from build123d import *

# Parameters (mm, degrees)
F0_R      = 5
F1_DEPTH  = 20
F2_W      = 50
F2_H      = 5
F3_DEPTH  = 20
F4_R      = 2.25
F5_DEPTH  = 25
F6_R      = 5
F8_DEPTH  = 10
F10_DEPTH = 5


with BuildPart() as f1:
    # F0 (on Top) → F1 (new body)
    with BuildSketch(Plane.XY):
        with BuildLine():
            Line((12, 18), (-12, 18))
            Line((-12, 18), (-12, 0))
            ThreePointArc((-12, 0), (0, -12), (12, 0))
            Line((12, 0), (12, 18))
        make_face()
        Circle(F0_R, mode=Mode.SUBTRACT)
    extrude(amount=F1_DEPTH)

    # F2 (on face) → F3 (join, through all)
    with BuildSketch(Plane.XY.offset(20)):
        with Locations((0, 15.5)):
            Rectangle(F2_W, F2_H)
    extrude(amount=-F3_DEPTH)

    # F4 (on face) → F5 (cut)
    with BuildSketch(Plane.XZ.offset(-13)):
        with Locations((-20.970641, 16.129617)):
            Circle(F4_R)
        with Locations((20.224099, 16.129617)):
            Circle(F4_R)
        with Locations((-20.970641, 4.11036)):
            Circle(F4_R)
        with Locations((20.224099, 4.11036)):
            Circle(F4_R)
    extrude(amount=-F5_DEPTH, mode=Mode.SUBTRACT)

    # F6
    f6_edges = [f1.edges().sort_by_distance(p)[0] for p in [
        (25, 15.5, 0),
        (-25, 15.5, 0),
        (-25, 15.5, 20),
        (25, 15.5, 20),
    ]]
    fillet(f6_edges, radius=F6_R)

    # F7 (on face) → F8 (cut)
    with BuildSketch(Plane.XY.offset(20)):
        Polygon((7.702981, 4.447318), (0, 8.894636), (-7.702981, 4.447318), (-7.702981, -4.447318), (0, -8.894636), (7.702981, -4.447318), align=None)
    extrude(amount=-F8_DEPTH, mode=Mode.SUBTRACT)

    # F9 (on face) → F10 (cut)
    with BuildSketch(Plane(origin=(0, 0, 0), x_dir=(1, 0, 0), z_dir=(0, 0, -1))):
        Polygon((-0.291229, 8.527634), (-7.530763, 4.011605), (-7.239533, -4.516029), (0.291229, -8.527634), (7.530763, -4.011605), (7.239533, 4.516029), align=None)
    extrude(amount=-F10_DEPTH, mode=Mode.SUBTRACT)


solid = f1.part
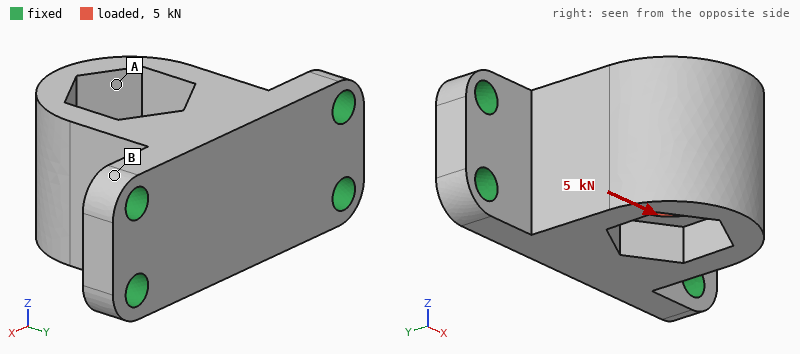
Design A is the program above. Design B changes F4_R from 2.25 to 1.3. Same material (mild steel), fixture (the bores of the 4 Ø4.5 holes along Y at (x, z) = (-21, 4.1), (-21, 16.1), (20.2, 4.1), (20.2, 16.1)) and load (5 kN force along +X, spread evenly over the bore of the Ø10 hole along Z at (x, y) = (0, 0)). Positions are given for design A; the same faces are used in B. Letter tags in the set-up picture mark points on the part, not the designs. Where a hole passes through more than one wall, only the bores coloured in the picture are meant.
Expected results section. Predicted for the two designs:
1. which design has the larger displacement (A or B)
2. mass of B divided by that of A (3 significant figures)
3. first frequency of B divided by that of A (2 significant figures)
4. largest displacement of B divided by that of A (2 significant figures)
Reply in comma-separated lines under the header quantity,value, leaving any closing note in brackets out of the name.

quantity,value
which design has the larger displacement,B
mass of B divided by that of A,1.02
first frequency of B divided by that of A,0.91
largest displacement of B divided by that of A,1.1
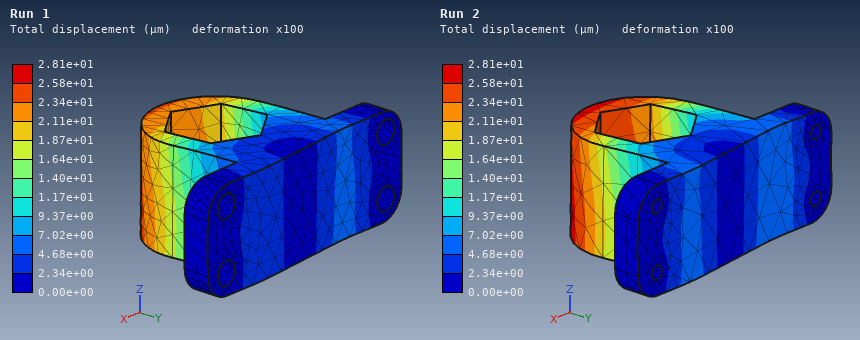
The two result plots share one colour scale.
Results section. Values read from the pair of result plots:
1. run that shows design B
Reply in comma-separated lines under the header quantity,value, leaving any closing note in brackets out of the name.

quantity,value
run that shows design B,Run 2
